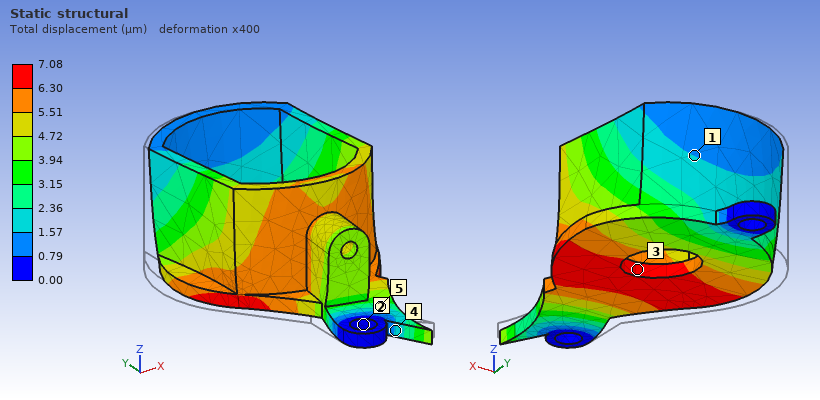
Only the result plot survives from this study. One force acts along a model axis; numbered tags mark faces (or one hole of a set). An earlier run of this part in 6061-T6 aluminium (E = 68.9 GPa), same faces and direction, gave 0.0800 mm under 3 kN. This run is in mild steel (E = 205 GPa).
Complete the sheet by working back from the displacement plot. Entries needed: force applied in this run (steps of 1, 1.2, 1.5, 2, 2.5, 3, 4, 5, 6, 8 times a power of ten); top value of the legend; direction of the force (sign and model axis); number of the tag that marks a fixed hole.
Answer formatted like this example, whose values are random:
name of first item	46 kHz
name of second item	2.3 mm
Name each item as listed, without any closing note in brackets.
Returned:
force applied in this run	800 N
top value of the legend	7.08 µm
direction of the force	+X
number of the tag that marks a fixed hole	2
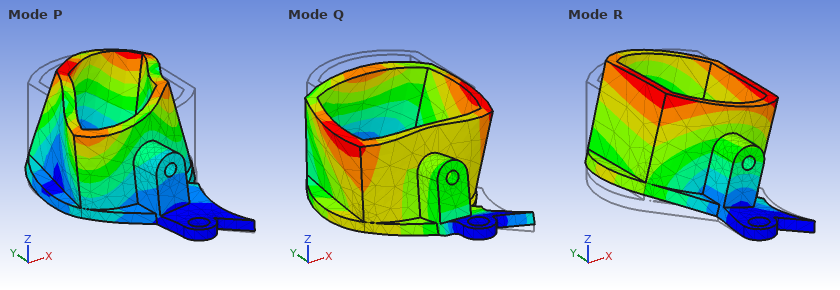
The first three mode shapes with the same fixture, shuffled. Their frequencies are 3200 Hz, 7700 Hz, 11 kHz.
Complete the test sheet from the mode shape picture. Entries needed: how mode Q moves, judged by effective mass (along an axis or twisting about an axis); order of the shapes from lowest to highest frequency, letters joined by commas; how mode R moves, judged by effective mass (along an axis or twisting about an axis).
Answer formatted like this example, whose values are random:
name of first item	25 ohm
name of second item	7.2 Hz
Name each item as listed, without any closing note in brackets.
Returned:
how mode Q moves, judged by effective mass	along Z
order of the shapes from lowest to highest frequency, letters joined by commas	R, Q, P
how mode R moves, judged by effective mass	along X
